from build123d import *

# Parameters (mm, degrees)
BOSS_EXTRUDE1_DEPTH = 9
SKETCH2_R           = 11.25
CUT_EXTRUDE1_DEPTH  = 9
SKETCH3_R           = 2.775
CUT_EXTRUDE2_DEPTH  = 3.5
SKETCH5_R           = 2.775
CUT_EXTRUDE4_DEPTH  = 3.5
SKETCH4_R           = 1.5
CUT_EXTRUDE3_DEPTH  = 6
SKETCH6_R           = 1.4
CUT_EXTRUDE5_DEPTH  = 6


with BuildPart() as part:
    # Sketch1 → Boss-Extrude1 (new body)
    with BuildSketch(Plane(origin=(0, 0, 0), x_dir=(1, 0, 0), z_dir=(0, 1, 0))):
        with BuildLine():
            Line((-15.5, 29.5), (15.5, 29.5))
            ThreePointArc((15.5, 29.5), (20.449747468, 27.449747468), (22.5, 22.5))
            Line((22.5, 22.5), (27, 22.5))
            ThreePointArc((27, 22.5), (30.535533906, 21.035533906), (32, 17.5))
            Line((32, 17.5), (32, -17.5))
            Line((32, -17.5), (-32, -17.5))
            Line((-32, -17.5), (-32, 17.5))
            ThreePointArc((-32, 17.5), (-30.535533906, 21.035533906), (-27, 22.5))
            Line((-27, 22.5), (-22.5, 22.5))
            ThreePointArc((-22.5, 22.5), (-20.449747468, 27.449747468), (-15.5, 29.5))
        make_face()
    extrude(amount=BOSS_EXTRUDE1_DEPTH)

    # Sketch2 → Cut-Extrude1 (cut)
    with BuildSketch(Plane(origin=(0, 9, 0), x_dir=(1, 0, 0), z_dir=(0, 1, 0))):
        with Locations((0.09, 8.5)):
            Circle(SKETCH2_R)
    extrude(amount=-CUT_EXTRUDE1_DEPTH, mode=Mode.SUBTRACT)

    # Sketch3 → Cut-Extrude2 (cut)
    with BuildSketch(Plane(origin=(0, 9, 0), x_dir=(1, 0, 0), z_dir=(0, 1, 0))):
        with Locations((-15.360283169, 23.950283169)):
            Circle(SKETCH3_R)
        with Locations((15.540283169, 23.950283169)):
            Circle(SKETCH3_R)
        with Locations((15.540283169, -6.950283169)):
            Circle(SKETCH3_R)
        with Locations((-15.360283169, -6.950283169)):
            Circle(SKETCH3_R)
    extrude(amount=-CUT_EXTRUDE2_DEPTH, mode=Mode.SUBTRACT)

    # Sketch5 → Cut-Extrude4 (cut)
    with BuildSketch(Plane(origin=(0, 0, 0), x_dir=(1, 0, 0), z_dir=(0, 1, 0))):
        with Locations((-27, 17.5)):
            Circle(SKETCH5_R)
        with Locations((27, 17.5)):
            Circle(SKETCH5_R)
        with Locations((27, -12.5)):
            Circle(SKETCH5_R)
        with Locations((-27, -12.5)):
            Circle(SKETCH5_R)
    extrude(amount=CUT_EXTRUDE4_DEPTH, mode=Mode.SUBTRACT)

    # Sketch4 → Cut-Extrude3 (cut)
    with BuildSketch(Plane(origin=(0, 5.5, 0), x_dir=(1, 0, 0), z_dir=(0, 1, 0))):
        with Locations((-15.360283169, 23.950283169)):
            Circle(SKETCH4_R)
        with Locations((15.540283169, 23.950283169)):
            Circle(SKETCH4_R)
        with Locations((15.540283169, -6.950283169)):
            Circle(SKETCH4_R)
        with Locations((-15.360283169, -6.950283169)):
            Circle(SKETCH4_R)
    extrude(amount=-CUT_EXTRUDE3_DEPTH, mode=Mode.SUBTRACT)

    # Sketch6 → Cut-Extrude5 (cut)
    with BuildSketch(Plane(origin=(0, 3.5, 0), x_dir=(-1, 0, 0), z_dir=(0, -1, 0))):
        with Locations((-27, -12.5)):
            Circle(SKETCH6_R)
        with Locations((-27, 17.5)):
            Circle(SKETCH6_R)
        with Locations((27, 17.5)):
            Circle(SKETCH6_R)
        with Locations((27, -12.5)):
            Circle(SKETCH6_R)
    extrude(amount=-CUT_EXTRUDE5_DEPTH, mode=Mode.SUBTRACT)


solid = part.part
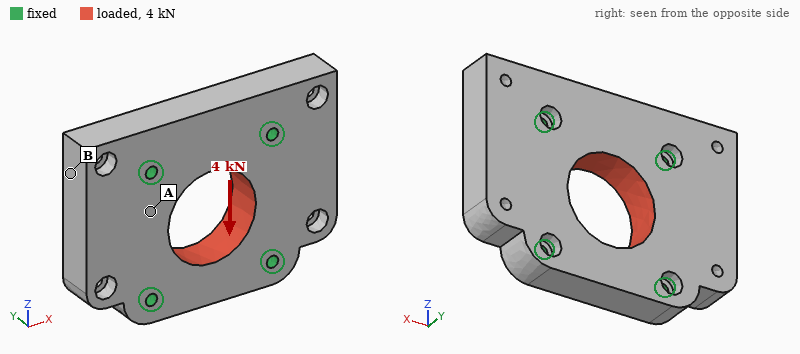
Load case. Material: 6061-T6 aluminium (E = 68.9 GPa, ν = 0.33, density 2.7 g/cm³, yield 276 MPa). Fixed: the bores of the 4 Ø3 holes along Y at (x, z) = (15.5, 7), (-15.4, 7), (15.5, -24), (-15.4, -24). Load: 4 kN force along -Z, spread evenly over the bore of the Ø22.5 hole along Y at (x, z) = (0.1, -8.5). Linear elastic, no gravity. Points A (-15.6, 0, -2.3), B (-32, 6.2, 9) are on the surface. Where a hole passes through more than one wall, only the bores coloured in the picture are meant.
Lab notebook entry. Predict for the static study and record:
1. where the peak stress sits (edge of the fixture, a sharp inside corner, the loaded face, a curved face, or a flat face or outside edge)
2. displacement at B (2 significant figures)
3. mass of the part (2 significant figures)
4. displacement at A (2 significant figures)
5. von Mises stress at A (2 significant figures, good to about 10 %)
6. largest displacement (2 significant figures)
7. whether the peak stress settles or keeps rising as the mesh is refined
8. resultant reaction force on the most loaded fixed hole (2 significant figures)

edge of the fixture
1.0 µm
57 g
1.3 µm
9.7 MPa
5.1 µm
keeps rising
1.0 kN
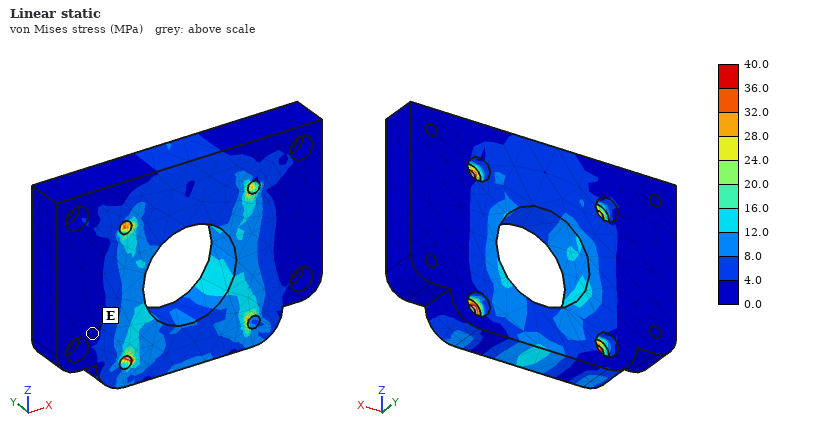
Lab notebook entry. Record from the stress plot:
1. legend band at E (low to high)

0.0 to 4.0 MPa
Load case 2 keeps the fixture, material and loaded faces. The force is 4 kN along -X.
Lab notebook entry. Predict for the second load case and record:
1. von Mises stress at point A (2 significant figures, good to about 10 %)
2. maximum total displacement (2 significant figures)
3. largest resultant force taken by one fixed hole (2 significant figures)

5.2 MPa
3.7 µm
1.0 kN
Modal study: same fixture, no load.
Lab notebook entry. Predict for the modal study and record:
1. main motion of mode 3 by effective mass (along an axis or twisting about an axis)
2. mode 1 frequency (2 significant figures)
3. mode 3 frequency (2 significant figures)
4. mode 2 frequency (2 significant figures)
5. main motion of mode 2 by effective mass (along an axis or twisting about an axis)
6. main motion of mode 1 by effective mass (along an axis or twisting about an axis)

twisting about X
13 kHz
20 kHz
14 kHz
twisting about Z
along Y
